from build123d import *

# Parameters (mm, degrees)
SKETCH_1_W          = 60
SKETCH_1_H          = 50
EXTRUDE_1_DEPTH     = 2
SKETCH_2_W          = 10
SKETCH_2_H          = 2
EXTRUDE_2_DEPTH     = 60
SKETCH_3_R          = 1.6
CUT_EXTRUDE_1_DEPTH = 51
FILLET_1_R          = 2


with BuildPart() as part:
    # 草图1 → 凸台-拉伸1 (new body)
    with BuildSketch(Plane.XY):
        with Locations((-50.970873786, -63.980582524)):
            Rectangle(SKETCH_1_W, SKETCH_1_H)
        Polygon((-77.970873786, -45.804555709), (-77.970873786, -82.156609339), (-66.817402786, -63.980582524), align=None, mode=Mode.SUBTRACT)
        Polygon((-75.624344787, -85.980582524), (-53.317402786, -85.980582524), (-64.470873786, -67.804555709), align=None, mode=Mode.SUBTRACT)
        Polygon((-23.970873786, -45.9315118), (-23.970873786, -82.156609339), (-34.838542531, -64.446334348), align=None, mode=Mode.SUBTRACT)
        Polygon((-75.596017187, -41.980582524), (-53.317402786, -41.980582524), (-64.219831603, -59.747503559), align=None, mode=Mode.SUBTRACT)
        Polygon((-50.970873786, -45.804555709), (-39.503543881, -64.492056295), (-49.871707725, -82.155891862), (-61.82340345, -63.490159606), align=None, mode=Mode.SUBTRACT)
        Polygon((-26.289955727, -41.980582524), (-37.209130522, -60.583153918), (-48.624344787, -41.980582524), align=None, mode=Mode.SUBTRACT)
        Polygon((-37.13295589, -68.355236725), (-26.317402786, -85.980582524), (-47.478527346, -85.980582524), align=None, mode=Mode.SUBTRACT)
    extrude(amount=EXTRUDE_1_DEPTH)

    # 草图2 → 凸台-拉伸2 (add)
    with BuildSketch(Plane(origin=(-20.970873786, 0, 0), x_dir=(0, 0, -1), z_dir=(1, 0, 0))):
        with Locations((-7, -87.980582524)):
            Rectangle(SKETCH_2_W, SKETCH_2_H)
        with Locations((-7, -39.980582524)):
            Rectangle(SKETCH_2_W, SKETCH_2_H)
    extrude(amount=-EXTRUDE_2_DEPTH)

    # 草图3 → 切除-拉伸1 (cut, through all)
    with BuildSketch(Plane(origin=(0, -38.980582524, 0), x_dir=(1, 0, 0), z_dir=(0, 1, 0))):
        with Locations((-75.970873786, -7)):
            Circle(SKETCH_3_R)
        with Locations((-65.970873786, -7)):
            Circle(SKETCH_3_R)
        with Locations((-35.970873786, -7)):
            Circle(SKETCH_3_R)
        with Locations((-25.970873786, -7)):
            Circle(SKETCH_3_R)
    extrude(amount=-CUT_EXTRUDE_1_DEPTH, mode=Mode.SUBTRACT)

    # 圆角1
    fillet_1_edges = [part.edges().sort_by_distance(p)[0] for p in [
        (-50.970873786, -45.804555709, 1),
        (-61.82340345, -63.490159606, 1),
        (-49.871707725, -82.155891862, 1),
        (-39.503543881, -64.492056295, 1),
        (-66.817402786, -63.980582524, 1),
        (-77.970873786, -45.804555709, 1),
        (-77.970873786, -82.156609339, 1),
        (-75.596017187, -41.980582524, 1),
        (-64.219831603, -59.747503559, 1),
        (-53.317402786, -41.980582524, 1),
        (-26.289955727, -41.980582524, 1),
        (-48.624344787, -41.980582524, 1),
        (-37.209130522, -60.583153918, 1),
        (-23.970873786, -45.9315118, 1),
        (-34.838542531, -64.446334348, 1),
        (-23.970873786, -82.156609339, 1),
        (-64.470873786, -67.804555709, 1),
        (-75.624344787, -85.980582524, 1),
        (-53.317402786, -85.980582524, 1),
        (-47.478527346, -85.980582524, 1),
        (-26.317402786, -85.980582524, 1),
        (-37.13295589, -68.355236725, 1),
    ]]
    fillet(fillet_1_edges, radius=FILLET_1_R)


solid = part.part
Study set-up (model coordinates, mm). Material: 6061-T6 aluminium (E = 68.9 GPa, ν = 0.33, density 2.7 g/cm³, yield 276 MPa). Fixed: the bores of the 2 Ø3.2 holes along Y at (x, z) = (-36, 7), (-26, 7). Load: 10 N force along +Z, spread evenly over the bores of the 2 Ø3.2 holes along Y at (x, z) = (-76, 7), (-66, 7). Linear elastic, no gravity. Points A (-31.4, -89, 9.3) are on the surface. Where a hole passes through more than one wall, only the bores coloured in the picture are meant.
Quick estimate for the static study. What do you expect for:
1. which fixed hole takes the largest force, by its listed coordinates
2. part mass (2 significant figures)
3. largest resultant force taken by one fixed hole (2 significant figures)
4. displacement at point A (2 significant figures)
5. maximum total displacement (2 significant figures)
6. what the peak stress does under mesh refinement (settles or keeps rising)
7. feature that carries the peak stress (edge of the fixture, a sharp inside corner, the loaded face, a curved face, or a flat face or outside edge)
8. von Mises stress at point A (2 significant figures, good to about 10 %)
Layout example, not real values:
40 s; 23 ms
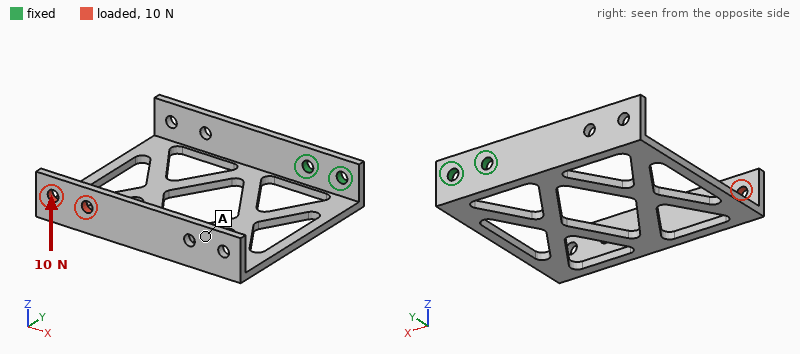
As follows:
(-36, 7); 14 g; 29 N; 0.54 mm; 0.86 mm; keeps rising; edge of the fixture; 3.8 MPa
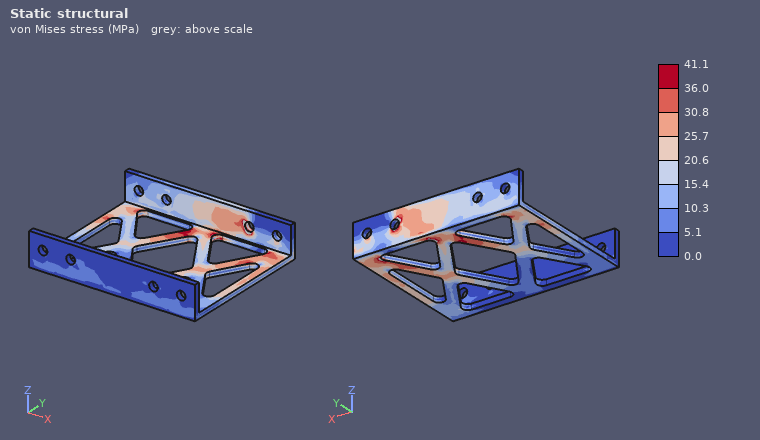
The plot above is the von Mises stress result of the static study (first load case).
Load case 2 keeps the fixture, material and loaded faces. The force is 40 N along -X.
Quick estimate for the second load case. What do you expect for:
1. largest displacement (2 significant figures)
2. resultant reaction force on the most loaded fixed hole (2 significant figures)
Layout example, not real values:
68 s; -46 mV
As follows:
0.41 mm; 120 N
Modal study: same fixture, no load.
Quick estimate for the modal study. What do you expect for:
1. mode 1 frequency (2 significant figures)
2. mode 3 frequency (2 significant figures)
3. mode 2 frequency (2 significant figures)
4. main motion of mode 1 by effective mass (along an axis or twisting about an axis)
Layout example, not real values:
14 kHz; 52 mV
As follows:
280 Hz; 880 Hz; 700 Hz; along Z
